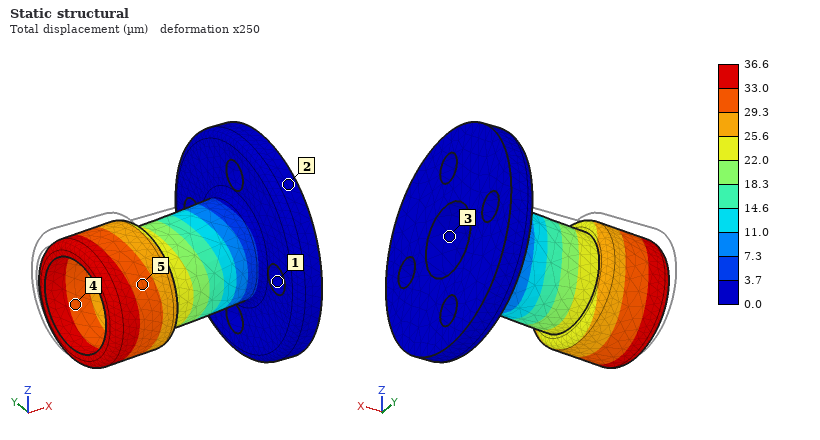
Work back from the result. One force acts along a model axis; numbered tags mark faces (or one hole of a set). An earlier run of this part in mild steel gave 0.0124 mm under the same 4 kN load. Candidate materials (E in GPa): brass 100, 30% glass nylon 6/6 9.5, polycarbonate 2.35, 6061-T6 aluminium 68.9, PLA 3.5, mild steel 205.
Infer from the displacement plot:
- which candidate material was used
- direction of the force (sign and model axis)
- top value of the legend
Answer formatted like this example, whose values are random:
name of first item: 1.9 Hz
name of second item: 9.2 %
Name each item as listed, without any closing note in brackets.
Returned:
which candidate material was used: 6061-T6 aluminium
direction of the force: -Y
top value of the legend: 36.6 µm
